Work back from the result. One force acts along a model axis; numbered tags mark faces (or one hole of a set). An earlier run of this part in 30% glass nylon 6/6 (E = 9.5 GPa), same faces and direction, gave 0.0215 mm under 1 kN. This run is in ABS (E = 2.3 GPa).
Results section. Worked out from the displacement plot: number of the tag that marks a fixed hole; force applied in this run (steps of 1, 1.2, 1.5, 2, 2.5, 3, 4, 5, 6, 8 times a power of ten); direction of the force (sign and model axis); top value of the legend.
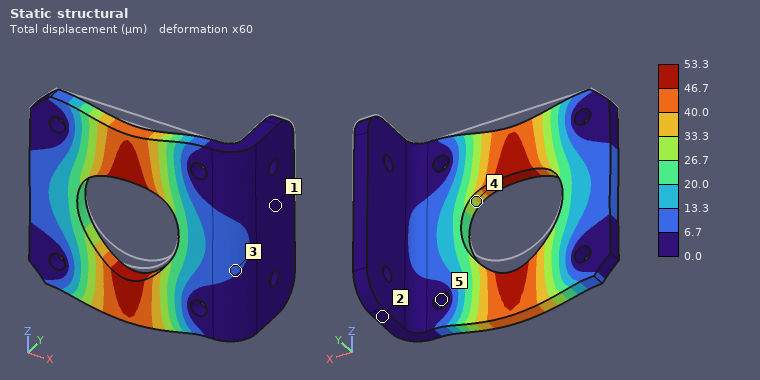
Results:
5
600 N
-Z
53.3 µm
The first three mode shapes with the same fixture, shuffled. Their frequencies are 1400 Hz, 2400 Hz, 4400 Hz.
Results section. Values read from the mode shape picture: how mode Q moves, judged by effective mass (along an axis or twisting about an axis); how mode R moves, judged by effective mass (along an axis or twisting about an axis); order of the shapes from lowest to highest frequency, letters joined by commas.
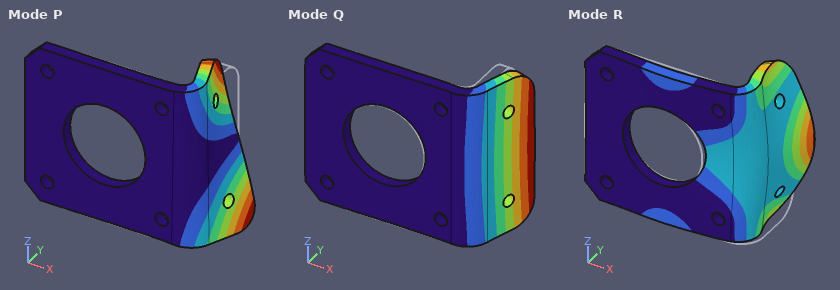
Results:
along X
along Y
Q, P, R
